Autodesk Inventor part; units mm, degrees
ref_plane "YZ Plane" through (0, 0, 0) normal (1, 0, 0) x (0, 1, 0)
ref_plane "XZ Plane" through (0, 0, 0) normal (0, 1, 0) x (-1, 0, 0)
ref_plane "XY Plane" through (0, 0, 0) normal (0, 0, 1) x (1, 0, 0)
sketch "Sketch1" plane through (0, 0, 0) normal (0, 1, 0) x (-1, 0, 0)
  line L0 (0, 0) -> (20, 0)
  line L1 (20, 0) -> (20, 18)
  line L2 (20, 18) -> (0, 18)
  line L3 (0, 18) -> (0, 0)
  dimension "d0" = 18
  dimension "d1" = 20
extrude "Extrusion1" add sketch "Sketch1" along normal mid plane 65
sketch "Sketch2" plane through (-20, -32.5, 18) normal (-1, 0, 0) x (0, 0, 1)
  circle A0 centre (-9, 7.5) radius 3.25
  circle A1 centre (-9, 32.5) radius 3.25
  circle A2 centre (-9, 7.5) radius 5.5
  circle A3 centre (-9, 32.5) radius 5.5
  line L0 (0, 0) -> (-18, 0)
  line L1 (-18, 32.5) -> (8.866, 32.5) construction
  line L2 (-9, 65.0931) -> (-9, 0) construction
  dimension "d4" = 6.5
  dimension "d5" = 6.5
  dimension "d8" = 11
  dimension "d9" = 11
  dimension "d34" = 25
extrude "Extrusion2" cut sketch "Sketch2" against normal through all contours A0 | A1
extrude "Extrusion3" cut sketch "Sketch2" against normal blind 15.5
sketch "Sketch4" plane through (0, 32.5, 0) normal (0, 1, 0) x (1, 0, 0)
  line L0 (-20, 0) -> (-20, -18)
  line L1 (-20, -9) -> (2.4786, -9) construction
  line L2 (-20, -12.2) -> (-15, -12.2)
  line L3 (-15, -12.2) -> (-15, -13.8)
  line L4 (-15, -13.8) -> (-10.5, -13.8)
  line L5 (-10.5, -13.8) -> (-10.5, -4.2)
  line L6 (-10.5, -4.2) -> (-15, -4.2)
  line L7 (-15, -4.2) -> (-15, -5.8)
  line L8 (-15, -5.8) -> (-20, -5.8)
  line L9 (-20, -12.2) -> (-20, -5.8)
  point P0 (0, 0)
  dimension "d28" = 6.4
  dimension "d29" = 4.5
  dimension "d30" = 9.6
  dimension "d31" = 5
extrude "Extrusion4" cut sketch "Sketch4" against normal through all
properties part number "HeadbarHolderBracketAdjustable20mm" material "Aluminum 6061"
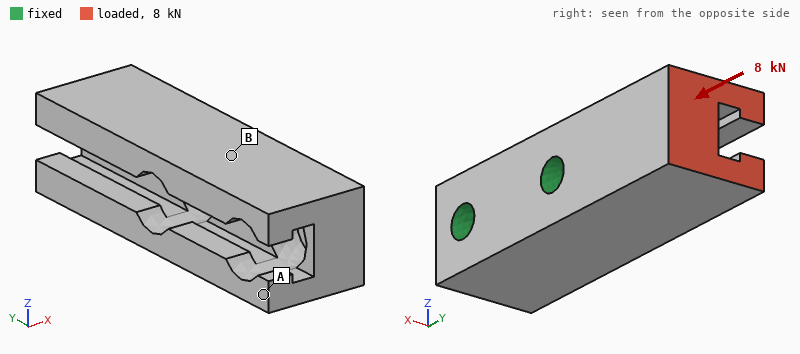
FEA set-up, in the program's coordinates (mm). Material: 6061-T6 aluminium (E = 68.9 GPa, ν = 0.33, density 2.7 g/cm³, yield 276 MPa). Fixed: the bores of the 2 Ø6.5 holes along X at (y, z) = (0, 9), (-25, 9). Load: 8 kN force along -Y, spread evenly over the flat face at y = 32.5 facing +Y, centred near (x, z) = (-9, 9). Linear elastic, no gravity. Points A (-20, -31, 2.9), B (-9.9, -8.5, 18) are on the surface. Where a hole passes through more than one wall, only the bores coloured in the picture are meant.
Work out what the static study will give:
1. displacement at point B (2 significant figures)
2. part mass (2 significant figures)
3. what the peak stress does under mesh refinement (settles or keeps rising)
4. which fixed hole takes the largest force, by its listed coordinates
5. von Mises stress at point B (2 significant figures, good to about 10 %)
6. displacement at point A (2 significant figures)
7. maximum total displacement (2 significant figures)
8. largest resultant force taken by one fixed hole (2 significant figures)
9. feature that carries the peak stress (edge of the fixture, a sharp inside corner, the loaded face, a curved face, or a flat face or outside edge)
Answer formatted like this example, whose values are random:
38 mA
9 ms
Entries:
8.2 µm
45 g
keeps rising
(0, 9)
34 MPa
13 µm
54 µm
5.9 kN
edge of the fixture
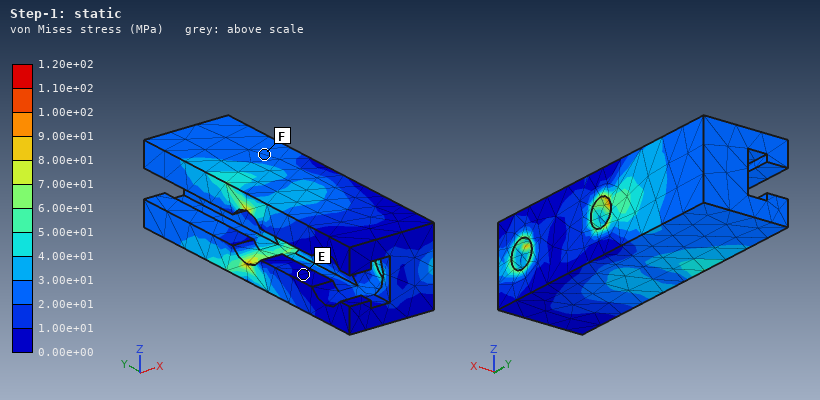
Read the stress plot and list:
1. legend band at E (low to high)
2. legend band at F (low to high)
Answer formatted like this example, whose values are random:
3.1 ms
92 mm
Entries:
0.00e+00 to 1.00e+01 MPa
2.00e+01 to 3.00e+01 MPa
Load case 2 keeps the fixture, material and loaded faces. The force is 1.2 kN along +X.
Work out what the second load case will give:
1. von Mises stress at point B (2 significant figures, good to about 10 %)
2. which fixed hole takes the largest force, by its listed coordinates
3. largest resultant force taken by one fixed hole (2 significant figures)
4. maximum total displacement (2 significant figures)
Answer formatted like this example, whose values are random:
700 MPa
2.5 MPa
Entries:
20 MPa
(0, 9)
2.7 kN
63 µm
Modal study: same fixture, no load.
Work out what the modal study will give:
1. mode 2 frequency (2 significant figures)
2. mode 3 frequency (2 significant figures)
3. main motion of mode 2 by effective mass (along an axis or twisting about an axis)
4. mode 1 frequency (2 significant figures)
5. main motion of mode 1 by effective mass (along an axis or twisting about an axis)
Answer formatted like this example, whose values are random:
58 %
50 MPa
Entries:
7800 Hz
10 kHz
along X
6400 Hz
along Z
